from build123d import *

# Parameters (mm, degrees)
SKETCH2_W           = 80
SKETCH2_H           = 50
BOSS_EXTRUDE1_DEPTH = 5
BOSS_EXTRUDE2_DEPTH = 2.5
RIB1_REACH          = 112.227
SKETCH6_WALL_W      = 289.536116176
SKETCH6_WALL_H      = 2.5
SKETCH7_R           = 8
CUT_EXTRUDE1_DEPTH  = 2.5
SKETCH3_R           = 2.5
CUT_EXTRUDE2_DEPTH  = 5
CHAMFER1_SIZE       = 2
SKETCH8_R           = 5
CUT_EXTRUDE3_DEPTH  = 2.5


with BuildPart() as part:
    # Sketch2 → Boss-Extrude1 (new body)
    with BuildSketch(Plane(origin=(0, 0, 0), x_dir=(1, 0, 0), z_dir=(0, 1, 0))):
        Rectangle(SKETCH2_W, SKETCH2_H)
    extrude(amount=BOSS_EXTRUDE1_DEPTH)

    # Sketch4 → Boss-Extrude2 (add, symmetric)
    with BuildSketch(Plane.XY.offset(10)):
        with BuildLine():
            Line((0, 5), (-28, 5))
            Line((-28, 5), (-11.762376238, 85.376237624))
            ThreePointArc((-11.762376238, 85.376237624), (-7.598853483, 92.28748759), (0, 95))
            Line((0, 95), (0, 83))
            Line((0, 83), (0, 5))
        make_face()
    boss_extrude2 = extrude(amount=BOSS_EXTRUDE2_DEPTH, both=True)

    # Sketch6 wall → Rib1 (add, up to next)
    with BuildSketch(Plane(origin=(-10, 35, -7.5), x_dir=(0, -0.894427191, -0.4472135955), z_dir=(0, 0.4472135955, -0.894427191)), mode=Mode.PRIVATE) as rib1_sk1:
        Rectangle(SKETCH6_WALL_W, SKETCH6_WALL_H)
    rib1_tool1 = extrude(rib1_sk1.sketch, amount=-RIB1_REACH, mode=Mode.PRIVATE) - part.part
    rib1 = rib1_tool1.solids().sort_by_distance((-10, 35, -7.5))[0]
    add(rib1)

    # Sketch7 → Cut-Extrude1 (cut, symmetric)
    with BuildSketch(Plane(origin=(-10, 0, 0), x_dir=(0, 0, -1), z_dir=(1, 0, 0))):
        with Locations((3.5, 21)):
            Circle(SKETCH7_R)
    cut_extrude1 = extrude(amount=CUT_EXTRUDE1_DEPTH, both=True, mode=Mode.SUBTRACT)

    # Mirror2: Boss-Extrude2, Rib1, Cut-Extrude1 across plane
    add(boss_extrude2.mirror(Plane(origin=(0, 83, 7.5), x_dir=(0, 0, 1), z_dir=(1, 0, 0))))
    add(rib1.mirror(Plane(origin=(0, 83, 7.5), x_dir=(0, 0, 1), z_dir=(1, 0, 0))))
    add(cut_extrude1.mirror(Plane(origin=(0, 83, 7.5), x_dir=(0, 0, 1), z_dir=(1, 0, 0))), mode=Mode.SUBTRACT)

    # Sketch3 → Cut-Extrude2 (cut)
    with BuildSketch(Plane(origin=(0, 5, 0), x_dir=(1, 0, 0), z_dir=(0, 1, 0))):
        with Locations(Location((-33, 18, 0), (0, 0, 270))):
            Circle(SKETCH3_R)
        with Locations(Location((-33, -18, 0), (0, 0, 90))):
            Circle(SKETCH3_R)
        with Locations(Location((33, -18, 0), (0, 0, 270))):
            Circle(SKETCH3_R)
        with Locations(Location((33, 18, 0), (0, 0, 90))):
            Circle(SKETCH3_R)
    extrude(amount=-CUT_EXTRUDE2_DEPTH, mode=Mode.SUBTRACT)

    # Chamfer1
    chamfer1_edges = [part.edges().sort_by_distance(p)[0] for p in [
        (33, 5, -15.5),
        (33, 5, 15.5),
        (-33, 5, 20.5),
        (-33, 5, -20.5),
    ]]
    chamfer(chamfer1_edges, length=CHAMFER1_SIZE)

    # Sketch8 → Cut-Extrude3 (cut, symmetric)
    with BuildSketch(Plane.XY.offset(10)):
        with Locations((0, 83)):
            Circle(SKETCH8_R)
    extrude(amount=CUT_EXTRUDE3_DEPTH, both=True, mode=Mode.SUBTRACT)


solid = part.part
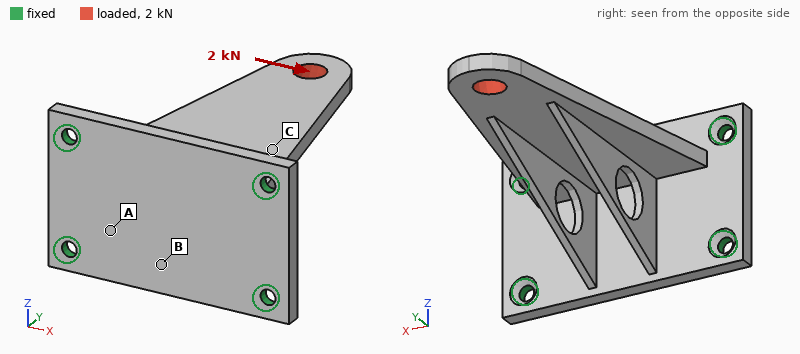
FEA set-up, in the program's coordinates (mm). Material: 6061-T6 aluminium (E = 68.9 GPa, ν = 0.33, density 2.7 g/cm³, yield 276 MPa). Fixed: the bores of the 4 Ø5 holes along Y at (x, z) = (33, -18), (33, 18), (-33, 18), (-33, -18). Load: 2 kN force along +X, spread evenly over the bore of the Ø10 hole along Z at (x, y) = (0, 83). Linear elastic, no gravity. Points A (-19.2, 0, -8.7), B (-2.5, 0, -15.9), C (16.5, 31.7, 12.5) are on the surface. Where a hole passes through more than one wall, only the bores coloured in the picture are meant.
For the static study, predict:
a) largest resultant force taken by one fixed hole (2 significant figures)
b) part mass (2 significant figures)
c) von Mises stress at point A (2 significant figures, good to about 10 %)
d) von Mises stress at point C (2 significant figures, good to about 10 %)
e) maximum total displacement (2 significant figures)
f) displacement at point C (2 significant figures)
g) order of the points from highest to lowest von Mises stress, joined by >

2.5 kN
110 g
25 MPa
45 MPa
0.32 mm
0.075 mm
C > A > B
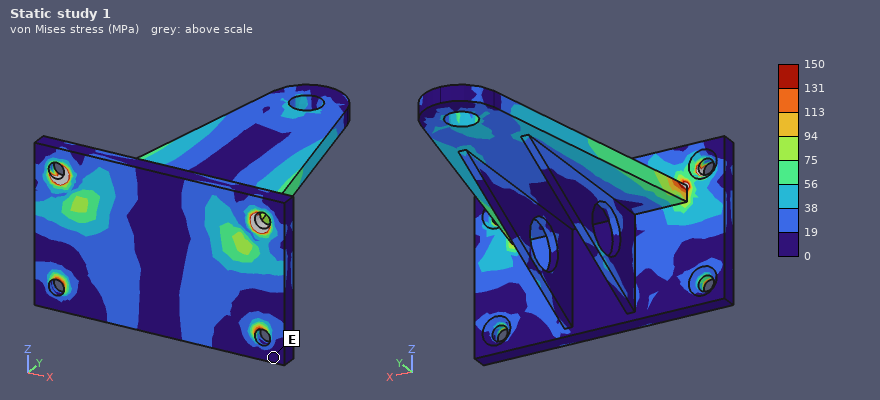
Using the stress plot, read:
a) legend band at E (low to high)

0 to 19 MPa
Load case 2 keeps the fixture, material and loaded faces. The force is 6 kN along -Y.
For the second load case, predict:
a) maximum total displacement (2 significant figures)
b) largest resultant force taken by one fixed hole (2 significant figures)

0.19 mm
2.9 kN
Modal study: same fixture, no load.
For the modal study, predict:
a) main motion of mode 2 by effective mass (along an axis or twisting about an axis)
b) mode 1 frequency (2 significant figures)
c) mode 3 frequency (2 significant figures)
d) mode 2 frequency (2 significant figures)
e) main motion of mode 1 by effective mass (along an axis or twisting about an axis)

along X
1500 Hz
4200 Hz
3700 Hz
along Z
